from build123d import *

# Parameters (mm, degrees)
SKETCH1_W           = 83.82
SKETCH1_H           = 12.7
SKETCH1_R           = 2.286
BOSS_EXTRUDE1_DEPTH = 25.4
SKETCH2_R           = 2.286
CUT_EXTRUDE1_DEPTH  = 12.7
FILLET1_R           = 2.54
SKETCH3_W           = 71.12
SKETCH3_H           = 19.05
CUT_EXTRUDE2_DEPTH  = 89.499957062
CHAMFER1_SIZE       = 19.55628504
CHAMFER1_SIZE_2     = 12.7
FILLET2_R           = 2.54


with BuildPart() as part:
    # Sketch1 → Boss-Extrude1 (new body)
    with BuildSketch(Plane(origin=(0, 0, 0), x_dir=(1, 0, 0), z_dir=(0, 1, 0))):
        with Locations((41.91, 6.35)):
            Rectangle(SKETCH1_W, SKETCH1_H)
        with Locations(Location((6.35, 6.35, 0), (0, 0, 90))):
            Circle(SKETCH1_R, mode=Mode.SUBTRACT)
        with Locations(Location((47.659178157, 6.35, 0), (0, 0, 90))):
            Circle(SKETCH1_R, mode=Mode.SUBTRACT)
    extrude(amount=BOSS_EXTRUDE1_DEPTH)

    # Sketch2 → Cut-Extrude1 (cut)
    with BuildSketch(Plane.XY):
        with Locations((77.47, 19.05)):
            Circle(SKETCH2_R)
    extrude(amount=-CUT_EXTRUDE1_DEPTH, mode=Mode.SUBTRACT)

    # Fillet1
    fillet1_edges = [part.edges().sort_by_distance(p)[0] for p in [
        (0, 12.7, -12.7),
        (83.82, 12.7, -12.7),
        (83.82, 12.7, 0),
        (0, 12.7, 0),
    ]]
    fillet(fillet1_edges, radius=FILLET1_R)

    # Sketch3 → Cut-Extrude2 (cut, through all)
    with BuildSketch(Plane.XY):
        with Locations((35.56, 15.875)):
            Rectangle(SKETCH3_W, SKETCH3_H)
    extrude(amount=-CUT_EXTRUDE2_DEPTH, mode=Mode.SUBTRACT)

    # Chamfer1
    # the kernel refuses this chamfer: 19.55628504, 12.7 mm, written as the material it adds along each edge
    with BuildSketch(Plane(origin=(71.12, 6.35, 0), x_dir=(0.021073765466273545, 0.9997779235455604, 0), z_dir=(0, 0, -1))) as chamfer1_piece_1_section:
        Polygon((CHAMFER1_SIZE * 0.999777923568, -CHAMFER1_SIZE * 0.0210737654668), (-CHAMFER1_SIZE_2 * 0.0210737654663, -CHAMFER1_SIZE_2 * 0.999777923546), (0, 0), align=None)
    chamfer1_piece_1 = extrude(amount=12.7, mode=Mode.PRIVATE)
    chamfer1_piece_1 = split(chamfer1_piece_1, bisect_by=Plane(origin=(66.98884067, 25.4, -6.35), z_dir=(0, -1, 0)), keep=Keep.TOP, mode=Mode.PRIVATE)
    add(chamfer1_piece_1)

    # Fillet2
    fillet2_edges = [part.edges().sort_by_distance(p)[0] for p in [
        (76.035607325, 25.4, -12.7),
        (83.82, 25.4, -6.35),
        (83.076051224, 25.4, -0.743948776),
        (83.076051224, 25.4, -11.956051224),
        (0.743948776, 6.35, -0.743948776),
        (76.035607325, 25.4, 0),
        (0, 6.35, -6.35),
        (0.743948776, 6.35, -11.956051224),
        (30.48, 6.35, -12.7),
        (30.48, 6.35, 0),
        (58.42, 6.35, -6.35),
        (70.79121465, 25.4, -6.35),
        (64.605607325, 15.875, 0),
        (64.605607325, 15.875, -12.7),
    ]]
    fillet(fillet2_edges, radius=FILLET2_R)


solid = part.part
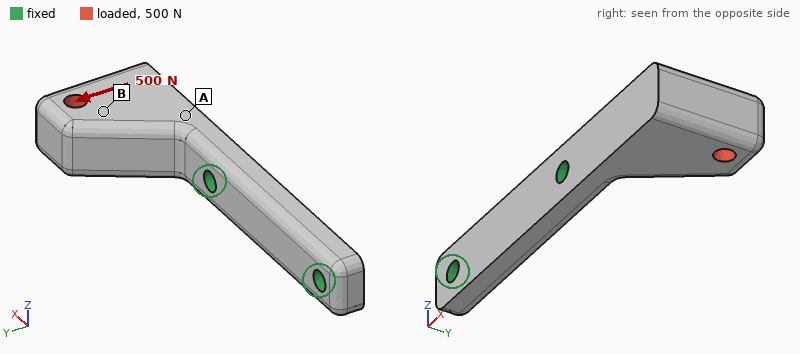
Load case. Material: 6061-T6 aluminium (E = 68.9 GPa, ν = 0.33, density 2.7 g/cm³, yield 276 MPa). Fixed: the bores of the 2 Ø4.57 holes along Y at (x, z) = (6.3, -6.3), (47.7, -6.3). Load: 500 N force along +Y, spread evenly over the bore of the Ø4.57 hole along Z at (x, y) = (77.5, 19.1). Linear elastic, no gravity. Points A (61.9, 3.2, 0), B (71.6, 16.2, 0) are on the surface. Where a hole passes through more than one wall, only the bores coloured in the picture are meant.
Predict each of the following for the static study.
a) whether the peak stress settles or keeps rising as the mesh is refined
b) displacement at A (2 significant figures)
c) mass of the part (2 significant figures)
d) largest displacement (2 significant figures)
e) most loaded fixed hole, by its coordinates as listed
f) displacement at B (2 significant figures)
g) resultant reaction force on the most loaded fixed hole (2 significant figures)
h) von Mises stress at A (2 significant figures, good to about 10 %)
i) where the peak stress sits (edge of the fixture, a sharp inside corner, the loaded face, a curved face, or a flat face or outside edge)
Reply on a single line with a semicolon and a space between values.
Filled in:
keeps rising; 0.064 mm; 29 g; 0.30 mm; (47.7, -6.3); 0.18 mm; 510 N; 40 MPa; edge of the fixture
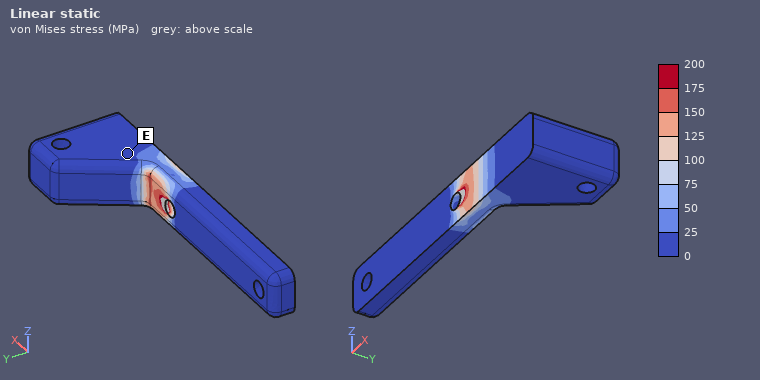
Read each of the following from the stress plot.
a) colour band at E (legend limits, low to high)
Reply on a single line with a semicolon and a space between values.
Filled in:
0 to 25 MPa
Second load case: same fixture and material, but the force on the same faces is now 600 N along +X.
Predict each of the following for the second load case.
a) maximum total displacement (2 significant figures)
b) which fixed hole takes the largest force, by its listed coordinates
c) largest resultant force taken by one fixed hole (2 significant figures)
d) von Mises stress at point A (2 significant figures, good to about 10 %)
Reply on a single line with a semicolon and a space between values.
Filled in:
0.25 mm; (47.7, -6.3); 600 N; 35 MPa
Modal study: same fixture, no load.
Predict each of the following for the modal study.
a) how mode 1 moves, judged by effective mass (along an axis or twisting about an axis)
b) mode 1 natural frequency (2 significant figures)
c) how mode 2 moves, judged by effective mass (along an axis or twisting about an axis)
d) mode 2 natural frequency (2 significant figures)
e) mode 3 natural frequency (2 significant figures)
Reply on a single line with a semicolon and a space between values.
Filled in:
along Y; 2000 Hz; along Z; 3000 Hz; 6900 Hz
